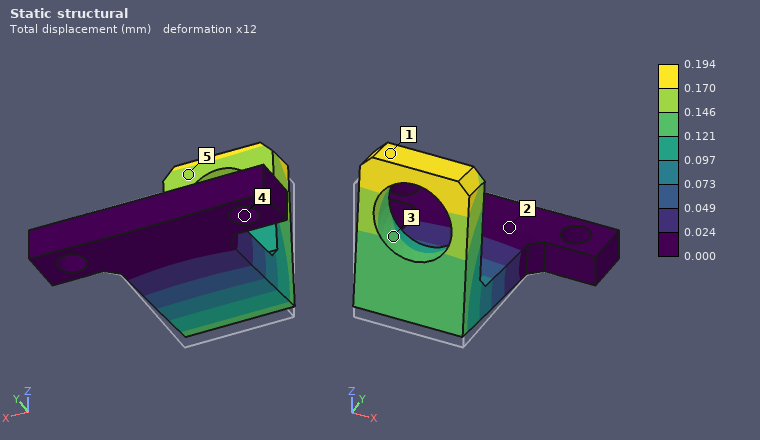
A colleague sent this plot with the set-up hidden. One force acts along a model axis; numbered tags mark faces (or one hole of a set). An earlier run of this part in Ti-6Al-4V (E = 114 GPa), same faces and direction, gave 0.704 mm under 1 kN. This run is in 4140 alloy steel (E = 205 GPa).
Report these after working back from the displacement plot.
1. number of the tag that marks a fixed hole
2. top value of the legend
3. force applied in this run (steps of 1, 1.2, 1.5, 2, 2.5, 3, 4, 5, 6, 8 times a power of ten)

4
0.194 mm
500 N
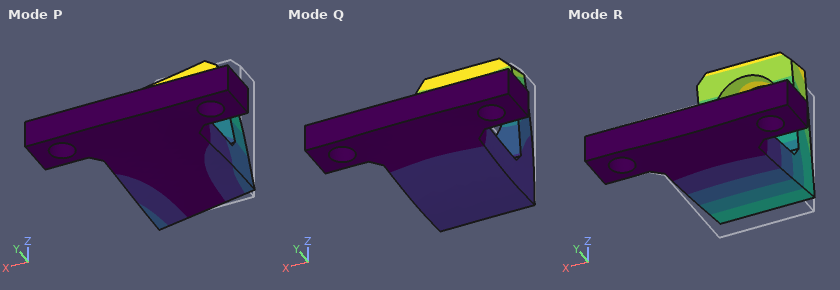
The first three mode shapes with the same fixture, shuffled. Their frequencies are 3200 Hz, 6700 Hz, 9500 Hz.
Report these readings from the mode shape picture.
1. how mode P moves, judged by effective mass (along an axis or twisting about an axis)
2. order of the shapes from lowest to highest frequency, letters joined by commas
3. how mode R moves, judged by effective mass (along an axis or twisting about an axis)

along X
R, P, Q
along Z
